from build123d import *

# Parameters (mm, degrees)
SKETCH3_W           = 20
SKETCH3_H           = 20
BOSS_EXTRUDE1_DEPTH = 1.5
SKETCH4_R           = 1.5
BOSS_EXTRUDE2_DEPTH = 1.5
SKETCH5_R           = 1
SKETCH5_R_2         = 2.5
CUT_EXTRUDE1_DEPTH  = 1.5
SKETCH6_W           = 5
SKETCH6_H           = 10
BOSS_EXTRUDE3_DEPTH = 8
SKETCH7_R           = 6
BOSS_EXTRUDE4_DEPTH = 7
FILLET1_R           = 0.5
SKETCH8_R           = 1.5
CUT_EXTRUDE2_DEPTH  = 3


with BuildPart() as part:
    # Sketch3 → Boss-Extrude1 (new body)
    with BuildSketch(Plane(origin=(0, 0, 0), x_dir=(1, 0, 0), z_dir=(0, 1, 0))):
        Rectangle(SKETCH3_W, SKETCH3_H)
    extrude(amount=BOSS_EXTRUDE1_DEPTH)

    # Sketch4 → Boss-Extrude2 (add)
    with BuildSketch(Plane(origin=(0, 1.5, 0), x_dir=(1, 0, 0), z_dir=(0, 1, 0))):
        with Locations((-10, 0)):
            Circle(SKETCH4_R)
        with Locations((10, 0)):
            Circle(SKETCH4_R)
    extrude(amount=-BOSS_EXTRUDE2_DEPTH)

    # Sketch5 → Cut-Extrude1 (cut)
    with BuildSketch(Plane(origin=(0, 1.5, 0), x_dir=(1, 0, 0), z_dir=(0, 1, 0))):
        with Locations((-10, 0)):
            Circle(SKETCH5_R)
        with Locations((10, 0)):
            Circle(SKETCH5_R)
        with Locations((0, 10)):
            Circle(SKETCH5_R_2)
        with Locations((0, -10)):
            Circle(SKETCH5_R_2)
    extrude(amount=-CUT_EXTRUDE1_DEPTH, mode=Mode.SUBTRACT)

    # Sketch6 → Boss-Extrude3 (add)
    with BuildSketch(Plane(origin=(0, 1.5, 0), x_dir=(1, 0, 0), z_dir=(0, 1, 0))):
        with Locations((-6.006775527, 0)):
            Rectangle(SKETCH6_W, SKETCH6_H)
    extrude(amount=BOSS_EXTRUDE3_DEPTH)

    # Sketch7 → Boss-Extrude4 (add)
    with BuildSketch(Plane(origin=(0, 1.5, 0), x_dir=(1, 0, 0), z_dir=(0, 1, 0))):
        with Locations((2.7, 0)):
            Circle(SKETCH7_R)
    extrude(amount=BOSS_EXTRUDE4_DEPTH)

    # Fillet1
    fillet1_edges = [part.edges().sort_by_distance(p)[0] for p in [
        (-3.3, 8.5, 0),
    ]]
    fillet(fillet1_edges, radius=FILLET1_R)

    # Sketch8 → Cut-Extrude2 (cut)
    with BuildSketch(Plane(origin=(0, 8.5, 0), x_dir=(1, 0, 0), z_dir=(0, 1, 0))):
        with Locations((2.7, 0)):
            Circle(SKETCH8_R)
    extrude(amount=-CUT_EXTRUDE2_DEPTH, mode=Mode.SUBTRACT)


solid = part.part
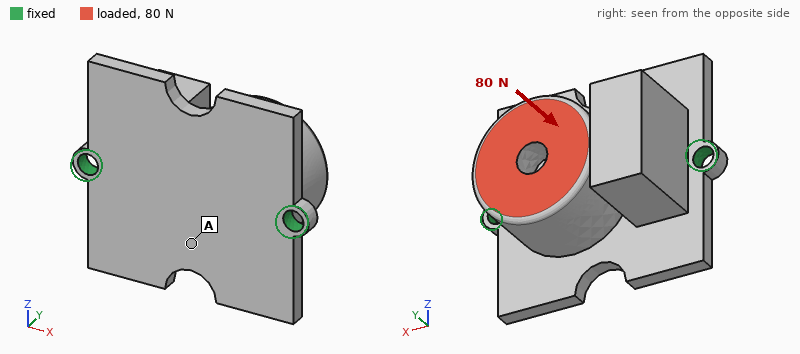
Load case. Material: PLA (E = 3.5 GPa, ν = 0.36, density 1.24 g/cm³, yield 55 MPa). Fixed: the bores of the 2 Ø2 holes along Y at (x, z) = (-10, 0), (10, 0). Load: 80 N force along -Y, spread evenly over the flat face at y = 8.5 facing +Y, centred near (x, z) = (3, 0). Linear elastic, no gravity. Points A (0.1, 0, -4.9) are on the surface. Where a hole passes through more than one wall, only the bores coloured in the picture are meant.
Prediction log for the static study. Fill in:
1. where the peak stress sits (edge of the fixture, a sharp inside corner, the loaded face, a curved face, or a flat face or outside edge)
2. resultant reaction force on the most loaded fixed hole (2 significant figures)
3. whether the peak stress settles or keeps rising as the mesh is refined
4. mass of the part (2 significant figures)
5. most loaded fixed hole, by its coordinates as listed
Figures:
edge of the fixture
55 N
keeps rising
2.2 g
(10, 0)
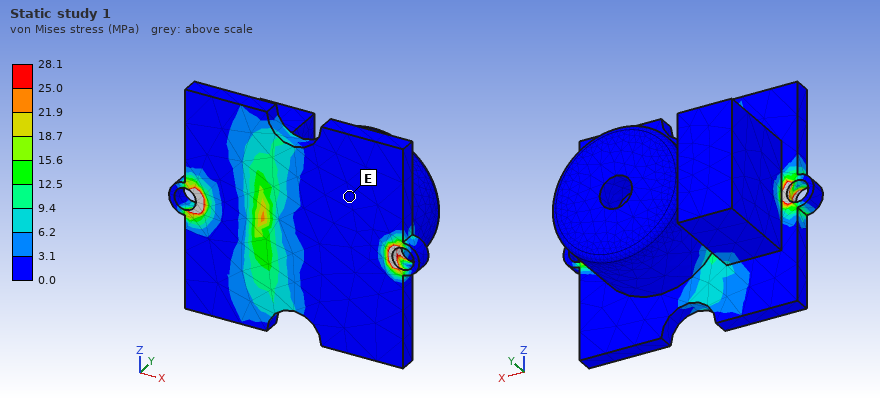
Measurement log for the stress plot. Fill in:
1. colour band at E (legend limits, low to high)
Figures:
0.0 to 3.1 MPa
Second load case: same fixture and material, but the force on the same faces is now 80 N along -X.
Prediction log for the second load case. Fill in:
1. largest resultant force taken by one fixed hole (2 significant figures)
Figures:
55 N
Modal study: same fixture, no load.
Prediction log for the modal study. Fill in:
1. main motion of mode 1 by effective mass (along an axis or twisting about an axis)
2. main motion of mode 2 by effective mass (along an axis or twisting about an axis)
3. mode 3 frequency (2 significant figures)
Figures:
along Z
along Y
7000 Hz
